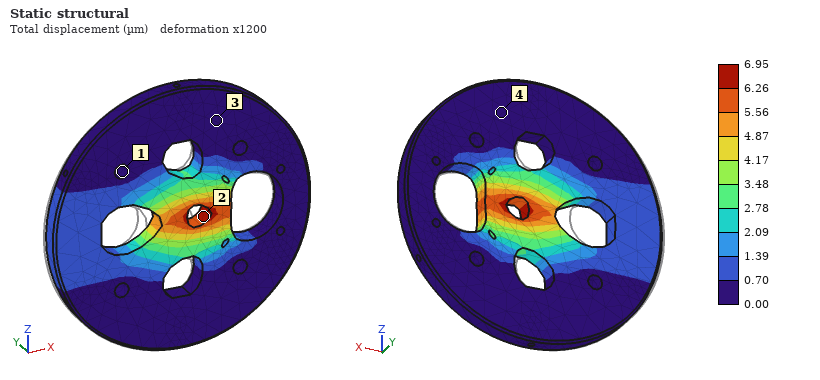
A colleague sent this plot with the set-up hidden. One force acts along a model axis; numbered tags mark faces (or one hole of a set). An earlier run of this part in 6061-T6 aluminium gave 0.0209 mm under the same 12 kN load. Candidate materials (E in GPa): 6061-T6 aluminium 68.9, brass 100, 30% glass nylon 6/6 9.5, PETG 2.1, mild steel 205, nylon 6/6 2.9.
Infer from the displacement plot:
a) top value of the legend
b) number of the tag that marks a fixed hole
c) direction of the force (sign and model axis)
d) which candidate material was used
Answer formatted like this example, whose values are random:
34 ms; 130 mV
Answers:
6.95 µm; 1; +X; mild steel
